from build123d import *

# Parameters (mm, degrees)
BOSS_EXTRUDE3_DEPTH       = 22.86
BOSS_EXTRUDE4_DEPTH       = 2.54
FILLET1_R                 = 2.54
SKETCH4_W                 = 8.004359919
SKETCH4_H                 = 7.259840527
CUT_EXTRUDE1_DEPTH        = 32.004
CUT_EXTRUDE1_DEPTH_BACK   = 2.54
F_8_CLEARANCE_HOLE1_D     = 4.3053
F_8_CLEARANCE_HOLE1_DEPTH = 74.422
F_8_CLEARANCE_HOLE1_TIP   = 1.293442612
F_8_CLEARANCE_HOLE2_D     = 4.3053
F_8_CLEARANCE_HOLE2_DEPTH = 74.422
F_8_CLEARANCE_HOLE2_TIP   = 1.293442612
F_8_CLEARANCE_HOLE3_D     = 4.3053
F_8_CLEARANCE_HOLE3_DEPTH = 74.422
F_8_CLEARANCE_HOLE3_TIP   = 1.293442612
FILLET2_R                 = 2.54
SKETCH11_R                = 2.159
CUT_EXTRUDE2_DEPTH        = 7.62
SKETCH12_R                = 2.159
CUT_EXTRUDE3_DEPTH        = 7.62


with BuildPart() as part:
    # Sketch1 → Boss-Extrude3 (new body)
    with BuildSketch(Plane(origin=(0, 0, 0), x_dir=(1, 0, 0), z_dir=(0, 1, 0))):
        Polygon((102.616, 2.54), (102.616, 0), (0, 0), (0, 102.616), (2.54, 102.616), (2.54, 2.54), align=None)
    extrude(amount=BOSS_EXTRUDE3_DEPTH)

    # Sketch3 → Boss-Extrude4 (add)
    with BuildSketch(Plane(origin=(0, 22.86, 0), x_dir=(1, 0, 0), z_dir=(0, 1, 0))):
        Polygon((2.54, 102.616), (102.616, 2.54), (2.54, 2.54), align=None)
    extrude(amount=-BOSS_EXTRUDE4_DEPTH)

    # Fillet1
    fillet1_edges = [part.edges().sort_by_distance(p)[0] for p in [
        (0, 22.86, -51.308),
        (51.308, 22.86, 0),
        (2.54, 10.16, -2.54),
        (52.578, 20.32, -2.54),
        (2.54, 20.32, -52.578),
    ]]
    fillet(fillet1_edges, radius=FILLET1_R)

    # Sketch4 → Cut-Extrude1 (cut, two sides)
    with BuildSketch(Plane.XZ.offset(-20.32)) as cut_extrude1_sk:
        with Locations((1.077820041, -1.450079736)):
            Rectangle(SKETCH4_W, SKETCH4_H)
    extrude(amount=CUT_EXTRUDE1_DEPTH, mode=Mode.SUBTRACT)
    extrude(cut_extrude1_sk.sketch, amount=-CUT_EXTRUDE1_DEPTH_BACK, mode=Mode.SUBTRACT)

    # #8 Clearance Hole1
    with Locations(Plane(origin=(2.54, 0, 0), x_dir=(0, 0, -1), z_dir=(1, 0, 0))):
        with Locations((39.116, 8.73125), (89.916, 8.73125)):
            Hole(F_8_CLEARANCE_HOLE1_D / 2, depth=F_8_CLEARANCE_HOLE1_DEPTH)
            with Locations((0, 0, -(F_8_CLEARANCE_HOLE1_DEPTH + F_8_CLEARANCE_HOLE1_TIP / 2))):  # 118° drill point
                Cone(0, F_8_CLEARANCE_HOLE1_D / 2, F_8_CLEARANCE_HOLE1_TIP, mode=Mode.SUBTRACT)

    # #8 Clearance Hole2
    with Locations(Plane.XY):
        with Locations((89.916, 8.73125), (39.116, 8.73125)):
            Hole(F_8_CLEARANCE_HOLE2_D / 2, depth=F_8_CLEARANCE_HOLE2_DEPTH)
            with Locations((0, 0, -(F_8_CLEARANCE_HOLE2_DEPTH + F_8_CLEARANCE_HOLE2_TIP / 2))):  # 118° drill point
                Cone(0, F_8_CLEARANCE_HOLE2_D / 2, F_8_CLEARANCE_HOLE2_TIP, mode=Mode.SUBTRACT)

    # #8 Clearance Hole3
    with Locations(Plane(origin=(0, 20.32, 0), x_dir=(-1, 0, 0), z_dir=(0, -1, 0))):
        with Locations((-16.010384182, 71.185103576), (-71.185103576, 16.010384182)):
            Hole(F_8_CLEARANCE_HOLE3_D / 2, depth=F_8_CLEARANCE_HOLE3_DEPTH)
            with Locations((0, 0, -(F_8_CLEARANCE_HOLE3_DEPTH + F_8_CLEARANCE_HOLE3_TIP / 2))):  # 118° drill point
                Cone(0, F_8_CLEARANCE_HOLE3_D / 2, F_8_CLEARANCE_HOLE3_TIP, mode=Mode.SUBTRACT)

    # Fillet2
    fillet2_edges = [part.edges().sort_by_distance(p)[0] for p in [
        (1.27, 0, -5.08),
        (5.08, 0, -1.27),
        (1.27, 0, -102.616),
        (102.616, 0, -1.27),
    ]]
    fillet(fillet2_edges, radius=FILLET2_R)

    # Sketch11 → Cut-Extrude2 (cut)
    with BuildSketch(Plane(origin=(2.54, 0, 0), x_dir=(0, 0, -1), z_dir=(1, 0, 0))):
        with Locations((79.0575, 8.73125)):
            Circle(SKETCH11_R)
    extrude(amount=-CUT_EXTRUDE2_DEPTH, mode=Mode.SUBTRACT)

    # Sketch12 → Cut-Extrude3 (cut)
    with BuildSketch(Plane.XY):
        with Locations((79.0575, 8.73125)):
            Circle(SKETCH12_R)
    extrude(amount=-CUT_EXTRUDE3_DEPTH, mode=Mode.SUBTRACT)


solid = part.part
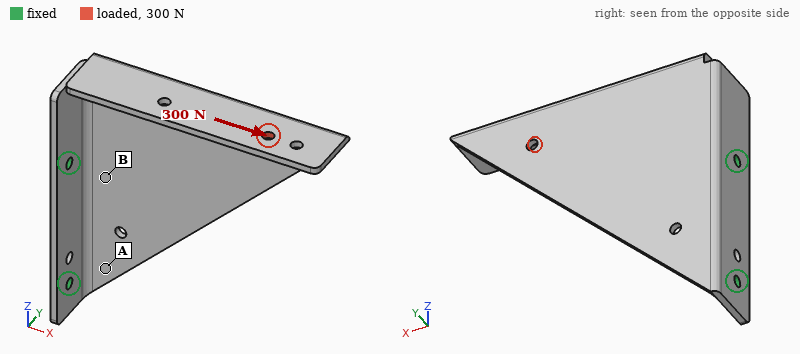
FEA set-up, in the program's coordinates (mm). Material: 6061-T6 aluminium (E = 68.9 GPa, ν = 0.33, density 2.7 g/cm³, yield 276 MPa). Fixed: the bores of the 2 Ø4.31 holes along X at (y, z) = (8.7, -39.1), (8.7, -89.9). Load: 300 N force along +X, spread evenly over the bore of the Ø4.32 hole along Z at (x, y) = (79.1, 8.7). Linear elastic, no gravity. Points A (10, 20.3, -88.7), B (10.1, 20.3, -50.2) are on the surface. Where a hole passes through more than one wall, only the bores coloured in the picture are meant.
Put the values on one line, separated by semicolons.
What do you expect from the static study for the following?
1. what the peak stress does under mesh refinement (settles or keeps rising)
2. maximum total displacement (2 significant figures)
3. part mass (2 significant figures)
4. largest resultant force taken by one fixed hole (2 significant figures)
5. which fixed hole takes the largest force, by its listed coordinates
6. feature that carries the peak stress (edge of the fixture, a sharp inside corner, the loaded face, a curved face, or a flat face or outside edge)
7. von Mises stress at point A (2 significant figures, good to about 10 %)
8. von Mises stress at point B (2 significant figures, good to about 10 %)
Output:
keeps rising; 1.6 mm; 64 g; 490 N; (8.7, -39.1); edge of the fixture; 17 MPa; 35 MPa
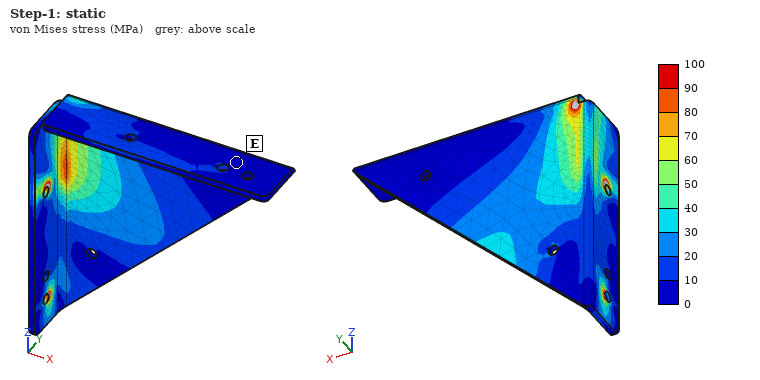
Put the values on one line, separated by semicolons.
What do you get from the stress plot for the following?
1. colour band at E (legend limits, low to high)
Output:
0 to 10 MPa
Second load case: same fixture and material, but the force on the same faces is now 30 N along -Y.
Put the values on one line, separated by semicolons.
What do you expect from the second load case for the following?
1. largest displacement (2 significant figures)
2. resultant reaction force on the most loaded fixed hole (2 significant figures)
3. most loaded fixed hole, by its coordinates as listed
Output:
1.5 mm; 52 N; (8.7, -39.1)
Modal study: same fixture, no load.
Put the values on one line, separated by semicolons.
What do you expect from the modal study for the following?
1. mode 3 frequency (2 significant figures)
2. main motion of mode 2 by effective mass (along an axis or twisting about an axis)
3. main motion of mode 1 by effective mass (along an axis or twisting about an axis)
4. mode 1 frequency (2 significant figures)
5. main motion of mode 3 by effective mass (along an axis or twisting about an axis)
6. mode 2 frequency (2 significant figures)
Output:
970 Hz; along Z; along Y; 210 Hz; along X; 890 Hz
